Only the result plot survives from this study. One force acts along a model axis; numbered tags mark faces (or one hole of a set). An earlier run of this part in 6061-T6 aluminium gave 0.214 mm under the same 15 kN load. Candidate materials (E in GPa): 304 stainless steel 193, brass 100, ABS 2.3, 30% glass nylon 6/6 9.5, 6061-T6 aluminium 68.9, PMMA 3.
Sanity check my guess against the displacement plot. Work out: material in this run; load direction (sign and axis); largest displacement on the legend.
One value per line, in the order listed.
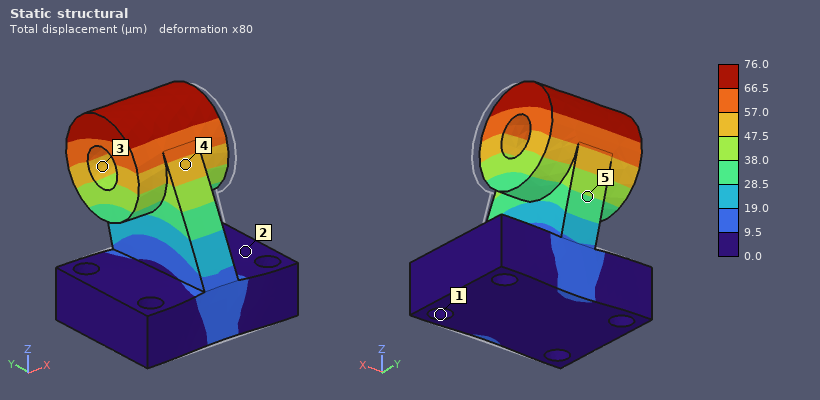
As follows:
304 stainless steel
+Y
76.0 µm
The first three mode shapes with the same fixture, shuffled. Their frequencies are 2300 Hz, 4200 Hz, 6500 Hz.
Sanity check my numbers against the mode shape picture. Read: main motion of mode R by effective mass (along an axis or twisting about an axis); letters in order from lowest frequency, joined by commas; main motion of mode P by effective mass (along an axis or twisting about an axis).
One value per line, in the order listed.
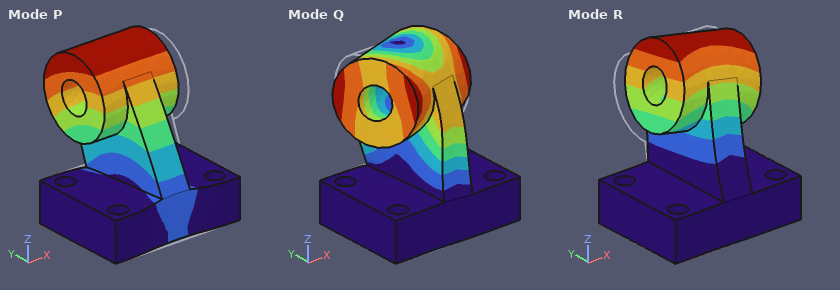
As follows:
along X
R, P, Q
along Y
